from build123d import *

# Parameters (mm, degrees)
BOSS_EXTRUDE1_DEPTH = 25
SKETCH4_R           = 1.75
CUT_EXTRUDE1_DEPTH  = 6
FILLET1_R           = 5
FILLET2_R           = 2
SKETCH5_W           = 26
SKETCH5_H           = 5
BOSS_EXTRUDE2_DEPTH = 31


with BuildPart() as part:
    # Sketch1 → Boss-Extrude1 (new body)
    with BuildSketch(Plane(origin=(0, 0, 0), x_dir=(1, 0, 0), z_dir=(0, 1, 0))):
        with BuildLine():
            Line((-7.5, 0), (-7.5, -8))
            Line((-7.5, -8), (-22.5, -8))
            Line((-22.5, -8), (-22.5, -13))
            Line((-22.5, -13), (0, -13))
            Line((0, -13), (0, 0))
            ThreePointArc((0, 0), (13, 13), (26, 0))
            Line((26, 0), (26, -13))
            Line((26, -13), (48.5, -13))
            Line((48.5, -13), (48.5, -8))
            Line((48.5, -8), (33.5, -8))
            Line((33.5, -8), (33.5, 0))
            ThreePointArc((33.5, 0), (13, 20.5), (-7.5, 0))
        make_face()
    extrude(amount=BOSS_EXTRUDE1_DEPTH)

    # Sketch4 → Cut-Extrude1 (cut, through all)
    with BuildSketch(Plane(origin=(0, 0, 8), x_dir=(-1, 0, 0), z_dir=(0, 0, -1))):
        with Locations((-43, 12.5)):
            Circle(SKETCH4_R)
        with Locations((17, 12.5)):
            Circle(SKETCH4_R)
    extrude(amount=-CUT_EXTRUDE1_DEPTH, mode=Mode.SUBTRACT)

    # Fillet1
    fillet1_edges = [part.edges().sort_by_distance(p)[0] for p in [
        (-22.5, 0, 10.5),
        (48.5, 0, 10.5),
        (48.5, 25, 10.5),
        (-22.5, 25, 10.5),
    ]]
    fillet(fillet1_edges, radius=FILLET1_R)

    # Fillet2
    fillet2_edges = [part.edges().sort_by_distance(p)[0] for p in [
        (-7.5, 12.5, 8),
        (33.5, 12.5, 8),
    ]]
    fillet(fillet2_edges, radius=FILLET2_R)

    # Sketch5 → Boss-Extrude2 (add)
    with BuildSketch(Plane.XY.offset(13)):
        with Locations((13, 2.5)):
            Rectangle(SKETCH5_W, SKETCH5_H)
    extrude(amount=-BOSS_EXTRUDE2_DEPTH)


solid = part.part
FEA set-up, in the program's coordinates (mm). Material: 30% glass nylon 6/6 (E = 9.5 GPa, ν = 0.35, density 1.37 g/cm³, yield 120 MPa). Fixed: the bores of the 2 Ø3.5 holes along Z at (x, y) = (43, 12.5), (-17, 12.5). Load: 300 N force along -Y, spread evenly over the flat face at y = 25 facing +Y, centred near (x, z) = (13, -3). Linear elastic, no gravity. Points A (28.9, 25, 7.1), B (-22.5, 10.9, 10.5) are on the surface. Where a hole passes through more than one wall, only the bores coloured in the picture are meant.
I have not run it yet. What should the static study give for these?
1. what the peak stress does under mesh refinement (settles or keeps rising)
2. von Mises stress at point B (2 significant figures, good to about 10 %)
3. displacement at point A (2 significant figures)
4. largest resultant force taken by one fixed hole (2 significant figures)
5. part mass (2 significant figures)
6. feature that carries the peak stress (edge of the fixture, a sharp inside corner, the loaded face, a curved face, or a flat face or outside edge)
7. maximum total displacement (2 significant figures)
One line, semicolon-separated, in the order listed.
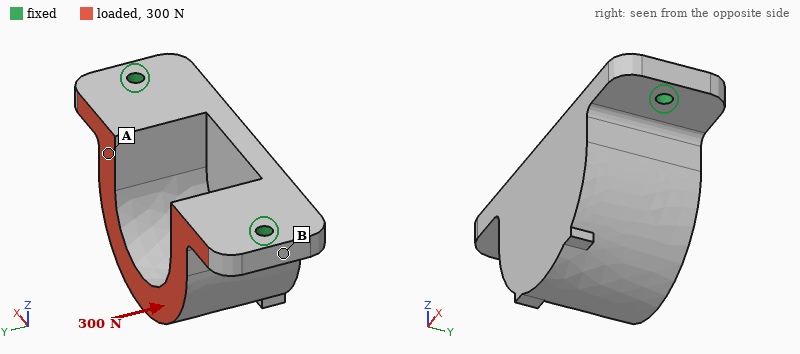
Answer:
keeps rising; 11 MPa; 0.091 mm; 190 N; 29 g; edge of the fixture; 0.24 mm
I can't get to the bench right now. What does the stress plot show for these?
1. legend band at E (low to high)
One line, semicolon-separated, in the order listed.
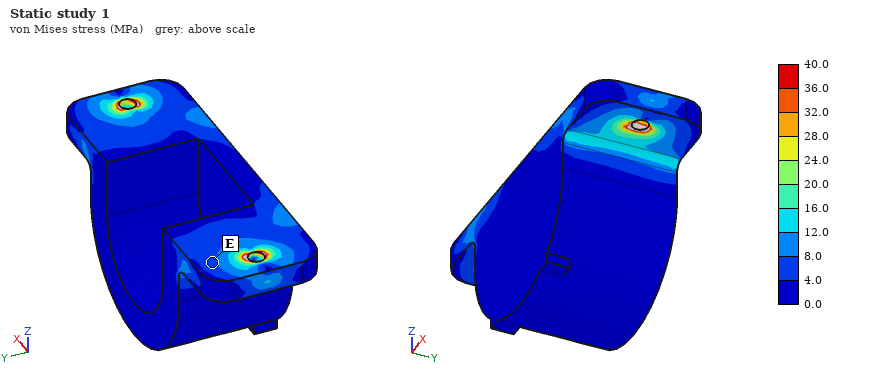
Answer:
4.0 to 8.0 MPa
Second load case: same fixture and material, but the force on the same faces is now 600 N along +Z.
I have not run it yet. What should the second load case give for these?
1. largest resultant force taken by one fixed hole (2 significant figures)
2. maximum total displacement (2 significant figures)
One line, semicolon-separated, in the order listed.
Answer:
340 N; 0.41 mm
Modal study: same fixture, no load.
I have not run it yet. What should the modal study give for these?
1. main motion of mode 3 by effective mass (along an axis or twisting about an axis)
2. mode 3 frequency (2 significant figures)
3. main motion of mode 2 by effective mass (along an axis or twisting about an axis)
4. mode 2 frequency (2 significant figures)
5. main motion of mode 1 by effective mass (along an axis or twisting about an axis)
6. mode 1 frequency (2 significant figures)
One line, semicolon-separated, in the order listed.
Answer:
along X; 4400 Hz; along Z; 3900 Hz; along Y; 1300 Hz
